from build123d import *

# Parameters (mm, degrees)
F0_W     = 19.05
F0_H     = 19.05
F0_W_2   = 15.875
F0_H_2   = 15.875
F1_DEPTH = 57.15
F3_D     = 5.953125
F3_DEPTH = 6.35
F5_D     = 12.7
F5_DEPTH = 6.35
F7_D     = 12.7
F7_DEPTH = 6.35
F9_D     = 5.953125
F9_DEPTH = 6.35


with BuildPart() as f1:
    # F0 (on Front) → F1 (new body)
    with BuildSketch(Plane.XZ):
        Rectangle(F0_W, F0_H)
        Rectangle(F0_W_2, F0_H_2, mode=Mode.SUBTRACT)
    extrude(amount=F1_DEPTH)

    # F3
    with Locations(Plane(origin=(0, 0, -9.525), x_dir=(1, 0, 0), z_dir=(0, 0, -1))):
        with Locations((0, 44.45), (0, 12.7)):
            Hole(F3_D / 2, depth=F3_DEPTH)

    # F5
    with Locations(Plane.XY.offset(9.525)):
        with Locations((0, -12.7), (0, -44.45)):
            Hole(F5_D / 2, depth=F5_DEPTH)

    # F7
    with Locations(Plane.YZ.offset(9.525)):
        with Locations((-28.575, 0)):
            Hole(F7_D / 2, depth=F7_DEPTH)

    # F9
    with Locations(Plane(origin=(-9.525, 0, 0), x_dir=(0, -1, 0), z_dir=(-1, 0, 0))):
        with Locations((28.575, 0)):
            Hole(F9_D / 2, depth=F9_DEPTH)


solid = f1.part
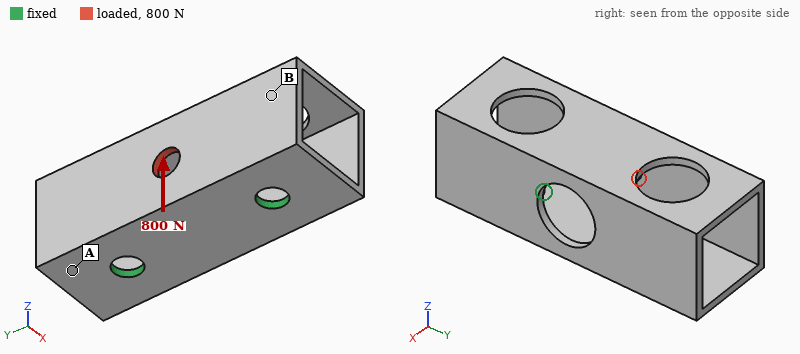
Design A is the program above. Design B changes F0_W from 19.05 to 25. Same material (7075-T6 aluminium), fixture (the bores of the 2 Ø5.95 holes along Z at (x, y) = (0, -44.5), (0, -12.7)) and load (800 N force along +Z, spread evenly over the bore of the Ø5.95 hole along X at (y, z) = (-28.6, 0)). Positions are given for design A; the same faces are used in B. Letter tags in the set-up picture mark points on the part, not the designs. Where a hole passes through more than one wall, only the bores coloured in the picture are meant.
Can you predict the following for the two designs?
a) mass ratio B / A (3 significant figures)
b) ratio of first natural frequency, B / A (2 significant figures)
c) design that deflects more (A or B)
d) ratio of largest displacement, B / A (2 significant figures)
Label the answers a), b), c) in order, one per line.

a) 2.07
b) 0.74
c) B
d) 1.2
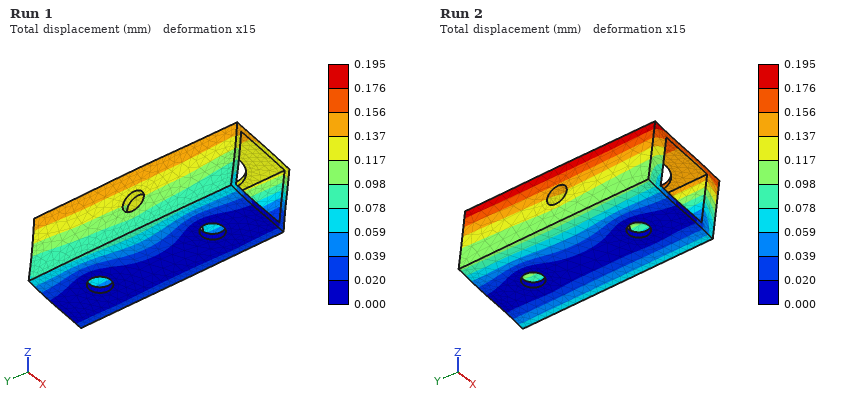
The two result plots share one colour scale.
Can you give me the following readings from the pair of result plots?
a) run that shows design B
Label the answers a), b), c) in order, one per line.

a) Run 2
